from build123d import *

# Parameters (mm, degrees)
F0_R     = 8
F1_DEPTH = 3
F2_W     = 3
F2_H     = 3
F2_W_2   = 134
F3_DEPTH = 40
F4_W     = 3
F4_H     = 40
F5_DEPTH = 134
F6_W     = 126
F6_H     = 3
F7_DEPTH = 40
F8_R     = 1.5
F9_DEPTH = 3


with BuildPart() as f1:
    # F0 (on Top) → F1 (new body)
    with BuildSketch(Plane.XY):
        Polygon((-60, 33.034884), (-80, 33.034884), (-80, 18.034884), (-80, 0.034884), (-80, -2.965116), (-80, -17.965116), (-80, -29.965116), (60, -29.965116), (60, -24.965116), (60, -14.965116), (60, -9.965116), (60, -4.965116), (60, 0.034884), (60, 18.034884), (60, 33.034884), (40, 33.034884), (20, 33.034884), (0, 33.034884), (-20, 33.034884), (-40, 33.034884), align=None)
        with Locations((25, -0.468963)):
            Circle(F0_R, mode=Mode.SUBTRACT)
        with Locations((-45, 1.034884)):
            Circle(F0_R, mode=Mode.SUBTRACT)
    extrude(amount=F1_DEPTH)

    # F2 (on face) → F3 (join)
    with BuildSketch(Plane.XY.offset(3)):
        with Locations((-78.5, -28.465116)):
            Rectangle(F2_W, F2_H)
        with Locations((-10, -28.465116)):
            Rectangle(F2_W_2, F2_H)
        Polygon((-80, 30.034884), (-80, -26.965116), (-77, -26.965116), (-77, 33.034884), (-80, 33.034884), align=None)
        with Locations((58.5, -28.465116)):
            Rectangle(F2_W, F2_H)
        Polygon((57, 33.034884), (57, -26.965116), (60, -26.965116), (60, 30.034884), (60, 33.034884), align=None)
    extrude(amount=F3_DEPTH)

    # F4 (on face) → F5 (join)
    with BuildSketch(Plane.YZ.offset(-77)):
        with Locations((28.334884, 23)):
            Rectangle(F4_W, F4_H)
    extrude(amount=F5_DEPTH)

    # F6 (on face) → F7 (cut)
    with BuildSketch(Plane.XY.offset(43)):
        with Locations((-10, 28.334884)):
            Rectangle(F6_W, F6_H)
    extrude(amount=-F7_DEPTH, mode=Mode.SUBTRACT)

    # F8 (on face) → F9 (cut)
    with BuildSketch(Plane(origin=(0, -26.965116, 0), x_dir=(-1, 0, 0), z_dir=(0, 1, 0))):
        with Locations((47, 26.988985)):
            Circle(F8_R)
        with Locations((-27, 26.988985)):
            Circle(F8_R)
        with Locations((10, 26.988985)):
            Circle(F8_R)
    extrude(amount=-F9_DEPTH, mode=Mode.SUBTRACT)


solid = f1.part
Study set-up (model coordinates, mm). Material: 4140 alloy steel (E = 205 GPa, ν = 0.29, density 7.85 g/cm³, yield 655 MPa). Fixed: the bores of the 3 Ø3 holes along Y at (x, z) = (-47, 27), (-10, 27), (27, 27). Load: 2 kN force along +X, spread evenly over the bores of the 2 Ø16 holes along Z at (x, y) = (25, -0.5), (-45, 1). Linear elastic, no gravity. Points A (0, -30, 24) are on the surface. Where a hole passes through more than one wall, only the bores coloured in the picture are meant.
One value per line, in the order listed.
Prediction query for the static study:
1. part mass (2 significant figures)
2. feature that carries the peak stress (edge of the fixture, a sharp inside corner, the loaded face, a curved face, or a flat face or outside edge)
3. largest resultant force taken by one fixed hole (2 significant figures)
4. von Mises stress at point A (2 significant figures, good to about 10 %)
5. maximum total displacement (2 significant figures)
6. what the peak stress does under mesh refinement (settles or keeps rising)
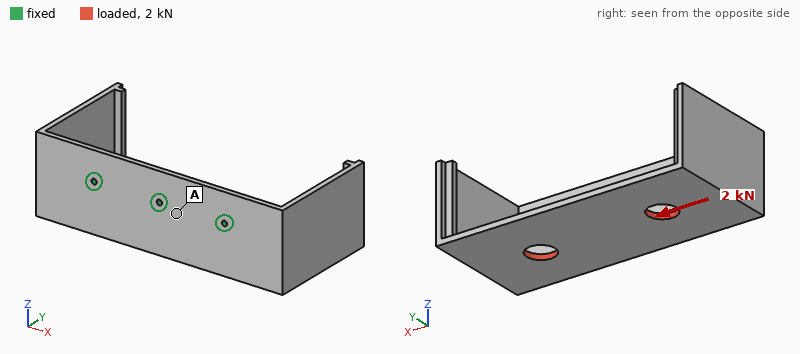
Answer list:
450 g
edge of the fixture
1.2 kN
32 MPa
0.43 mm
keeps rising
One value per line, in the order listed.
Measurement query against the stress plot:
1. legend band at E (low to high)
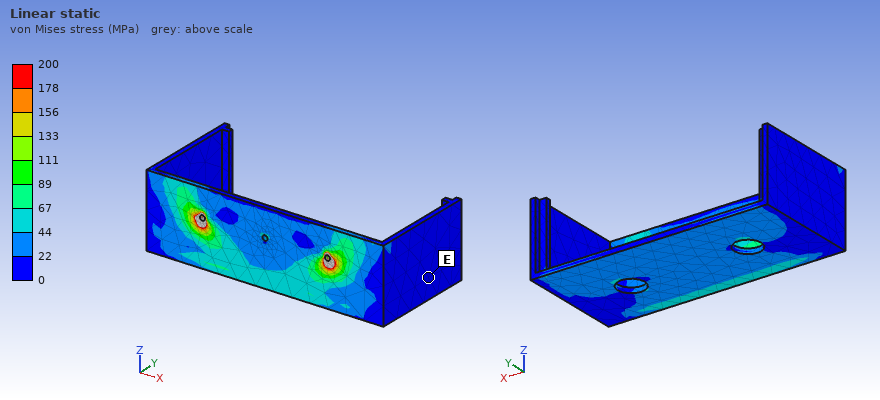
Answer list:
0 to 22 MPa
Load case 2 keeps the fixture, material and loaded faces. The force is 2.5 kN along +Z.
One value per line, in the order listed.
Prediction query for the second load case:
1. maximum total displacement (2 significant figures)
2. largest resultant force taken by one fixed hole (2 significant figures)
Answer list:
1.9 mm
1.1 kN
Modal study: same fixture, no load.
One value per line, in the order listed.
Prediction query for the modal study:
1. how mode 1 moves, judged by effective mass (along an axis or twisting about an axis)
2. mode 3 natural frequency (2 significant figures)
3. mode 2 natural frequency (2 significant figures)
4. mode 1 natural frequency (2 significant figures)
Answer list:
along Z
900 Hz
480 Hz
380 Hz
